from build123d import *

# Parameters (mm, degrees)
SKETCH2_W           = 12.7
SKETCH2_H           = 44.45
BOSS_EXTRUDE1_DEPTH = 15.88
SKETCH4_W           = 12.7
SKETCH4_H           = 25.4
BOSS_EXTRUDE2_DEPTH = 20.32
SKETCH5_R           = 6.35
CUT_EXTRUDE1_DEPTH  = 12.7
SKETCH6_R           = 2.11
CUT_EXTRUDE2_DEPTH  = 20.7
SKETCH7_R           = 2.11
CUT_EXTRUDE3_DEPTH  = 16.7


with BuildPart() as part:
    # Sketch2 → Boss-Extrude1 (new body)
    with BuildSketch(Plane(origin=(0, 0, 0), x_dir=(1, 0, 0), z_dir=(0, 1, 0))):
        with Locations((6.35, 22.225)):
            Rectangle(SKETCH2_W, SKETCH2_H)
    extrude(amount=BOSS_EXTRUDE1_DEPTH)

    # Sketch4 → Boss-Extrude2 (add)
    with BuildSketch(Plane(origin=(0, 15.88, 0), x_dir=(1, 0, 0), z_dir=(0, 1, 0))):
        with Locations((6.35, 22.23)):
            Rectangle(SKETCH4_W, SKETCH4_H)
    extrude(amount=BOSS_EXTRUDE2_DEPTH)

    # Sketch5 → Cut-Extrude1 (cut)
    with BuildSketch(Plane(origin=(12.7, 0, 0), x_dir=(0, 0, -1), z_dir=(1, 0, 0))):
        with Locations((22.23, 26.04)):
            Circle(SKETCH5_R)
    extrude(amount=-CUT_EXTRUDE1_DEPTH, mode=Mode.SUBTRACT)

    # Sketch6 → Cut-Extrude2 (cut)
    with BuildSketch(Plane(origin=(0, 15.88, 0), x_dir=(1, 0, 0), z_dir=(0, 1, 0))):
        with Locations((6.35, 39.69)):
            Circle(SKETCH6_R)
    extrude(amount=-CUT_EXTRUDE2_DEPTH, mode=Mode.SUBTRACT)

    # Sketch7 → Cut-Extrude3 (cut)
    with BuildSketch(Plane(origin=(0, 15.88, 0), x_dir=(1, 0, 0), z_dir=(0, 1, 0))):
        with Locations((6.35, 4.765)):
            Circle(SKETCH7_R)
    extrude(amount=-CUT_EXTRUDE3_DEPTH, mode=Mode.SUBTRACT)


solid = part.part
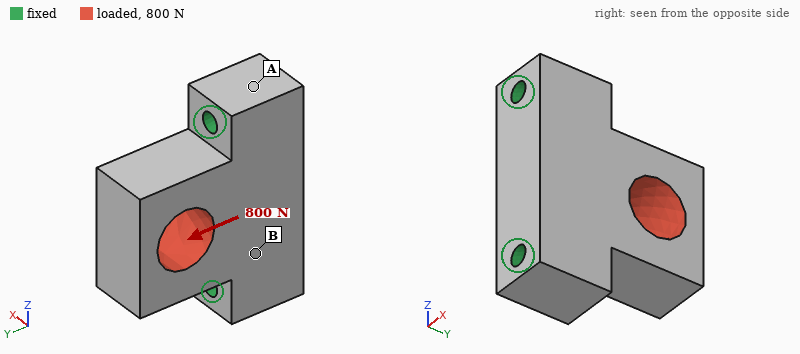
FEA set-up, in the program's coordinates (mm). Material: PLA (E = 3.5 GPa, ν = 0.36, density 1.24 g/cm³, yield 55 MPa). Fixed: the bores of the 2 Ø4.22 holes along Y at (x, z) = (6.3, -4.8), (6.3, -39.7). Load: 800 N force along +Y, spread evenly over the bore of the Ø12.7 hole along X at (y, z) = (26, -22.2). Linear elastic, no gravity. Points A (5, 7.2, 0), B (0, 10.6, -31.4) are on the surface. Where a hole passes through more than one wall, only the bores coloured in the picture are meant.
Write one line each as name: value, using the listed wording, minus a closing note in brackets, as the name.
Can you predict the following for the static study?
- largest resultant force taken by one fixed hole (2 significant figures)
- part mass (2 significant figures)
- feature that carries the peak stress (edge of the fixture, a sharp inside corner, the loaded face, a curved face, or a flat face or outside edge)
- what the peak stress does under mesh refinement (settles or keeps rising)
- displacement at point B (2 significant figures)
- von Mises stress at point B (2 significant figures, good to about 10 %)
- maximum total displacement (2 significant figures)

largest resultant force taken by one fixed hole: 420 N
part mass: 17 g
feature that carries the peak stress: edge of the fixture
what the peak stress does under mesh refinement: keeps rising
displacement at point B: 14 µm
von Mises stress at point B: 2.4 MPa
maximum total displacement: 46 µm
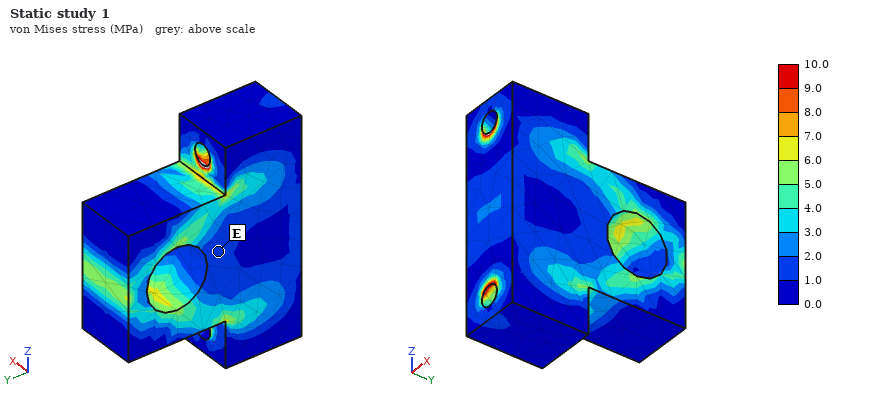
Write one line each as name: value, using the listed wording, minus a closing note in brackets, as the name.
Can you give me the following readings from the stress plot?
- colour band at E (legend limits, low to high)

colour band at E: 1.0 to 2.0 MPa
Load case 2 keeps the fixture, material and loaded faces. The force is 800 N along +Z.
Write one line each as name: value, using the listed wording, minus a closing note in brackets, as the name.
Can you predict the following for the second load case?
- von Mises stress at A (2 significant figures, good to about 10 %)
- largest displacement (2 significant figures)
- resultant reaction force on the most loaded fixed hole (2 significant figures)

von Mises stress at A: 1.2 MPa
largest displacement: 0.14 mm
resultant reaction force on the most loaded fixed hole: 570 N
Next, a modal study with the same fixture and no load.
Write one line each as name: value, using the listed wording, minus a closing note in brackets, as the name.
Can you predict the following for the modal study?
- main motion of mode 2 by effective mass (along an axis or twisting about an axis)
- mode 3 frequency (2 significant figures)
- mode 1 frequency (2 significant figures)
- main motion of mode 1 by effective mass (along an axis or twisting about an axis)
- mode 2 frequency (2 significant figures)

main motion of mode 2 by effective mass: along Z
mode 3 frequency: 6600 Hz
mode 1 frequency: 3200 Hz
main motion of mode 1 by effective mass: along X
mode 2 frequency: 5500 Hz
